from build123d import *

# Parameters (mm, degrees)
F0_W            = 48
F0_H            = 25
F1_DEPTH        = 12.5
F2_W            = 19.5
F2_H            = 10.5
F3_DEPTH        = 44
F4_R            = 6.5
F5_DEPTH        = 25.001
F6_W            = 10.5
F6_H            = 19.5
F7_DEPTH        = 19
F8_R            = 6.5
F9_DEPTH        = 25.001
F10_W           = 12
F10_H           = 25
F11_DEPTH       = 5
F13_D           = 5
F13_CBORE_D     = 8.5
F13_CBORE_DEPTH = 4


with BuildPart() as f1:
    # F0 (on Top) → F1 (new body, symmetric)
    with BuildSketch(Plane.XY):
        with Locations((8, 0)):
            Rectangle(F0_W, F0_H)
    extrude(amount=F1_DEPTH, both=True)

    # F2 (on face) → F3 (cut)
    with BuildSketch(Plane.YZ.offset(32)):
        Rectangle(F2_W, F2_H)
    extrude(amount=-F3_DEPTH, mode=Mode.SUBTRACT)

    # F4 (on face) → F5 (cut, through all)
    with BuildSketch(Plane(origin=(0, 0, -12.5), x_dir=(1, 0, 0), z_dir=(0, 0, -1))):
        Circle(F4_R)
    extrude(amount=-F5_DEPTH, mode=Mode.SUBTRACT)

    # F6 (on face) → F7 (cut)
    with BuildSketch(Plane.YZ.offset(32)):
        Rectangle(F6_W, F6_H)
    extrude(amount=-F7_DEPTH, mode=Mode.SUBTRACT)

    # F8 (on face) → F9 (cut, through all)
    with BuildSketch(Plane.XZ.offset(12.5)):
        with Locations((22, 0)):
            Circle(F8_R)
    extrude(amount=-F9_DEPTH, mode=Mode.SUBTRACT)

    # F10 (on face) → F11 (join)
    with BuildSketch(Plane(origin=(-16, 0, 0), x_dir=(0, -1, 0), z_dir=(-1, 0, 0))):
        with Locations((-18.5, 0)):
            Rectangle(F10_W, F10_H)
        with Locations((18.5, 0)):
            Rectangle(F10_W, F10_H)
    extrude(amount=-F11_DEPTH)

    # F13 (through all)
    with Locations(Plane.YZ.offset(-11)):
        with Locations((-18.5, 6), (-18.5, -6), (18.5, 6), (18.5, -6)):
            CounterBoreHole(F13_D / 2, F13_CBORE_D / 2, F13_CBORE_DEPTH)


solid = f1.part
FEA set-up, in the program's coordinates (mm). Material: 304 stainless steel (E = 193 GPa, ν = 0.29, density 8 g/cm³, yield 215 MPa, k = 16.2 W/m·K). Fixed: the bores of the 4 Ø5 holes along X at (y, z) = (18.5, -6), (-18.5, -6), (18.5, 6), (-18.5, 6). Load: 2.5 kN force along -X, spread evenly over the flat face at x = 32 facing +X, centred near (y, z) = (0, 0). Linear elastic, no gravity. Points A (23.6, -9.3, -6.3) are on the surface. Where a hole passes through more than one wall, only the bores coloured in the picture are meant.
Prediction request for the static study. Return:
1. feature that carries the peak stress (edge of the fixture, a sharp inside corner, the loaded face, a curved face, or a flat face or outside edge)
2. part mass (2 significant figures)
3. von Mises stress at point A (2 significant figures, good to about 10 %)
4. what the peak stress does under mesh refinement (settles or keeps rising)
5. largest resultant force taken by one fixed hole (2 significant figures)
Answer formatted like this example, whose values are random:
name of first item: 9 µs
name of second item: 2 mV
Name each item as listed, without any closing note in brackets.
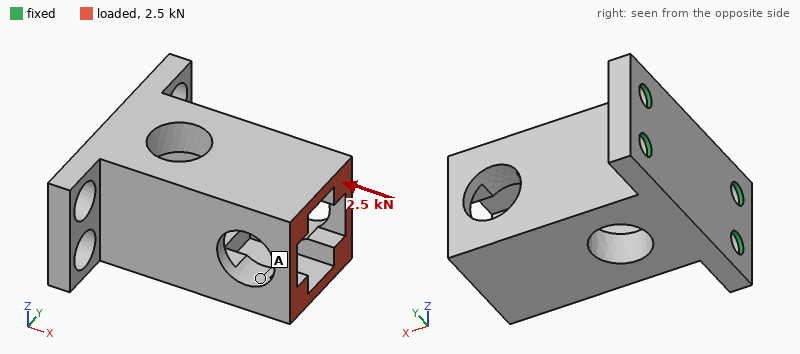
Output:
feature that carries the peak stress: edge of the fixture
part mass: 150 g
von Mises stress at point A: 29 MPa
what the peak stress does under mesh refinement: keeps rising
largest resultant force taken by one fixed hole: 810 N
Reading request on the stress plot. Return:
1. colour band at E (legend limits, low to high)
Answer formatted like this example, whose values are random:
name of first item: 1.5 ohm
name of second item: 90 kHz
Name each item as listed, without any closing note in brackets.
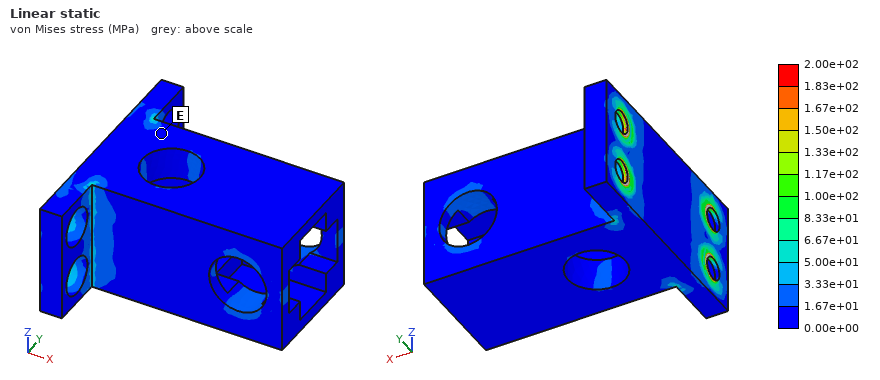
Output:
colour band at E: 0.00e+00 to 1.67e+01 MPa
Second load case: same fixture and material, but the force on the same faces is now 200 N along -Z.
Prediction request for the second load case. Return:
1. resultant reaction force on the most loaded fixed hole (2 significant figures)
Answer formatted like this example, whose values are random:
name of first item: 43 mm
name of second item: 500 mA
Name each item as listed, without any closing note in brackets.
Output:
resultant reaction force on the most loaded fixed hole: 390 N
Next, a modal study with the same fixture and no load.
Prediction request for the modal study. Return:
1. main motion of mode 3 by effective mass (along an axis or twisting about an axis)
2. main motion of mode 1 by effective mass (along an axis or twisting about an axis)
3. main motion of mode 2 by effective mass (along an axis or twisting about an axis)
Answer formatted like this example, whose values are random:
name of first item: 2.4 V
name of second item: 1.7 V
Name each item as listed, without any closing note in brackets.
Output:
main motion of mode 3 by effective mass: along X
main motion of mode 1 by effective mass: along Z
main motion of mode 2 by effective mass: along Y
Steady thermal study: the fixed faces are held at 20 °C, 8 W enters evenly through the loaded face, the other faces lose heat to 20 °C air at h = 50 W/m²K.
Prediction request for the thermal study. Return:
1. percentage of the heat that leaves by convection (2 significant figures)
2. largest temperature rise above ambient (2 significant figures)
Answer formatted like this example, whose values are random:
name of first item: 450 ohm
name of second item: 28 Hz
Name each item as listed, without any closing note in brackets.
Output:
percentage of the heat that leaves by convection: 86 %
largest temperature rise above ambient: 45 K
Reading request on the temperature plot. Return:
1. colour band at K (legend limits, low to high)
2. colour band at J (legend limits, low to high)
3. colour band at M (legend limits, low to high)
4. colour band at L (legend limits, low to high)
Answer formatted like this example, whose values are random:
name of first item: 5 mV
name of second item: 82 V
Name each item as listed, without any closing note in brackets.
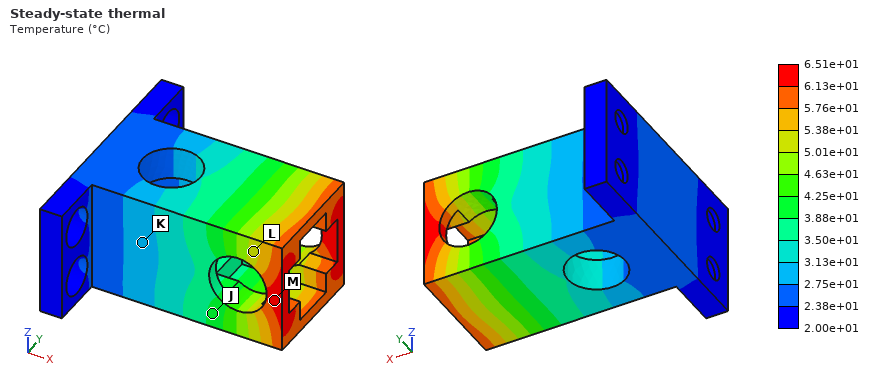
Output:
colour band at K: 2.75e+01 to 3.13e+01 °C
colour band at J: 3.88e+01 to 4.25e+01 °C
colour band at M: 6.13e+01 to 6.51e+01 °C
colour band at L: 5.01e+01 to 5.38e+01 °C
